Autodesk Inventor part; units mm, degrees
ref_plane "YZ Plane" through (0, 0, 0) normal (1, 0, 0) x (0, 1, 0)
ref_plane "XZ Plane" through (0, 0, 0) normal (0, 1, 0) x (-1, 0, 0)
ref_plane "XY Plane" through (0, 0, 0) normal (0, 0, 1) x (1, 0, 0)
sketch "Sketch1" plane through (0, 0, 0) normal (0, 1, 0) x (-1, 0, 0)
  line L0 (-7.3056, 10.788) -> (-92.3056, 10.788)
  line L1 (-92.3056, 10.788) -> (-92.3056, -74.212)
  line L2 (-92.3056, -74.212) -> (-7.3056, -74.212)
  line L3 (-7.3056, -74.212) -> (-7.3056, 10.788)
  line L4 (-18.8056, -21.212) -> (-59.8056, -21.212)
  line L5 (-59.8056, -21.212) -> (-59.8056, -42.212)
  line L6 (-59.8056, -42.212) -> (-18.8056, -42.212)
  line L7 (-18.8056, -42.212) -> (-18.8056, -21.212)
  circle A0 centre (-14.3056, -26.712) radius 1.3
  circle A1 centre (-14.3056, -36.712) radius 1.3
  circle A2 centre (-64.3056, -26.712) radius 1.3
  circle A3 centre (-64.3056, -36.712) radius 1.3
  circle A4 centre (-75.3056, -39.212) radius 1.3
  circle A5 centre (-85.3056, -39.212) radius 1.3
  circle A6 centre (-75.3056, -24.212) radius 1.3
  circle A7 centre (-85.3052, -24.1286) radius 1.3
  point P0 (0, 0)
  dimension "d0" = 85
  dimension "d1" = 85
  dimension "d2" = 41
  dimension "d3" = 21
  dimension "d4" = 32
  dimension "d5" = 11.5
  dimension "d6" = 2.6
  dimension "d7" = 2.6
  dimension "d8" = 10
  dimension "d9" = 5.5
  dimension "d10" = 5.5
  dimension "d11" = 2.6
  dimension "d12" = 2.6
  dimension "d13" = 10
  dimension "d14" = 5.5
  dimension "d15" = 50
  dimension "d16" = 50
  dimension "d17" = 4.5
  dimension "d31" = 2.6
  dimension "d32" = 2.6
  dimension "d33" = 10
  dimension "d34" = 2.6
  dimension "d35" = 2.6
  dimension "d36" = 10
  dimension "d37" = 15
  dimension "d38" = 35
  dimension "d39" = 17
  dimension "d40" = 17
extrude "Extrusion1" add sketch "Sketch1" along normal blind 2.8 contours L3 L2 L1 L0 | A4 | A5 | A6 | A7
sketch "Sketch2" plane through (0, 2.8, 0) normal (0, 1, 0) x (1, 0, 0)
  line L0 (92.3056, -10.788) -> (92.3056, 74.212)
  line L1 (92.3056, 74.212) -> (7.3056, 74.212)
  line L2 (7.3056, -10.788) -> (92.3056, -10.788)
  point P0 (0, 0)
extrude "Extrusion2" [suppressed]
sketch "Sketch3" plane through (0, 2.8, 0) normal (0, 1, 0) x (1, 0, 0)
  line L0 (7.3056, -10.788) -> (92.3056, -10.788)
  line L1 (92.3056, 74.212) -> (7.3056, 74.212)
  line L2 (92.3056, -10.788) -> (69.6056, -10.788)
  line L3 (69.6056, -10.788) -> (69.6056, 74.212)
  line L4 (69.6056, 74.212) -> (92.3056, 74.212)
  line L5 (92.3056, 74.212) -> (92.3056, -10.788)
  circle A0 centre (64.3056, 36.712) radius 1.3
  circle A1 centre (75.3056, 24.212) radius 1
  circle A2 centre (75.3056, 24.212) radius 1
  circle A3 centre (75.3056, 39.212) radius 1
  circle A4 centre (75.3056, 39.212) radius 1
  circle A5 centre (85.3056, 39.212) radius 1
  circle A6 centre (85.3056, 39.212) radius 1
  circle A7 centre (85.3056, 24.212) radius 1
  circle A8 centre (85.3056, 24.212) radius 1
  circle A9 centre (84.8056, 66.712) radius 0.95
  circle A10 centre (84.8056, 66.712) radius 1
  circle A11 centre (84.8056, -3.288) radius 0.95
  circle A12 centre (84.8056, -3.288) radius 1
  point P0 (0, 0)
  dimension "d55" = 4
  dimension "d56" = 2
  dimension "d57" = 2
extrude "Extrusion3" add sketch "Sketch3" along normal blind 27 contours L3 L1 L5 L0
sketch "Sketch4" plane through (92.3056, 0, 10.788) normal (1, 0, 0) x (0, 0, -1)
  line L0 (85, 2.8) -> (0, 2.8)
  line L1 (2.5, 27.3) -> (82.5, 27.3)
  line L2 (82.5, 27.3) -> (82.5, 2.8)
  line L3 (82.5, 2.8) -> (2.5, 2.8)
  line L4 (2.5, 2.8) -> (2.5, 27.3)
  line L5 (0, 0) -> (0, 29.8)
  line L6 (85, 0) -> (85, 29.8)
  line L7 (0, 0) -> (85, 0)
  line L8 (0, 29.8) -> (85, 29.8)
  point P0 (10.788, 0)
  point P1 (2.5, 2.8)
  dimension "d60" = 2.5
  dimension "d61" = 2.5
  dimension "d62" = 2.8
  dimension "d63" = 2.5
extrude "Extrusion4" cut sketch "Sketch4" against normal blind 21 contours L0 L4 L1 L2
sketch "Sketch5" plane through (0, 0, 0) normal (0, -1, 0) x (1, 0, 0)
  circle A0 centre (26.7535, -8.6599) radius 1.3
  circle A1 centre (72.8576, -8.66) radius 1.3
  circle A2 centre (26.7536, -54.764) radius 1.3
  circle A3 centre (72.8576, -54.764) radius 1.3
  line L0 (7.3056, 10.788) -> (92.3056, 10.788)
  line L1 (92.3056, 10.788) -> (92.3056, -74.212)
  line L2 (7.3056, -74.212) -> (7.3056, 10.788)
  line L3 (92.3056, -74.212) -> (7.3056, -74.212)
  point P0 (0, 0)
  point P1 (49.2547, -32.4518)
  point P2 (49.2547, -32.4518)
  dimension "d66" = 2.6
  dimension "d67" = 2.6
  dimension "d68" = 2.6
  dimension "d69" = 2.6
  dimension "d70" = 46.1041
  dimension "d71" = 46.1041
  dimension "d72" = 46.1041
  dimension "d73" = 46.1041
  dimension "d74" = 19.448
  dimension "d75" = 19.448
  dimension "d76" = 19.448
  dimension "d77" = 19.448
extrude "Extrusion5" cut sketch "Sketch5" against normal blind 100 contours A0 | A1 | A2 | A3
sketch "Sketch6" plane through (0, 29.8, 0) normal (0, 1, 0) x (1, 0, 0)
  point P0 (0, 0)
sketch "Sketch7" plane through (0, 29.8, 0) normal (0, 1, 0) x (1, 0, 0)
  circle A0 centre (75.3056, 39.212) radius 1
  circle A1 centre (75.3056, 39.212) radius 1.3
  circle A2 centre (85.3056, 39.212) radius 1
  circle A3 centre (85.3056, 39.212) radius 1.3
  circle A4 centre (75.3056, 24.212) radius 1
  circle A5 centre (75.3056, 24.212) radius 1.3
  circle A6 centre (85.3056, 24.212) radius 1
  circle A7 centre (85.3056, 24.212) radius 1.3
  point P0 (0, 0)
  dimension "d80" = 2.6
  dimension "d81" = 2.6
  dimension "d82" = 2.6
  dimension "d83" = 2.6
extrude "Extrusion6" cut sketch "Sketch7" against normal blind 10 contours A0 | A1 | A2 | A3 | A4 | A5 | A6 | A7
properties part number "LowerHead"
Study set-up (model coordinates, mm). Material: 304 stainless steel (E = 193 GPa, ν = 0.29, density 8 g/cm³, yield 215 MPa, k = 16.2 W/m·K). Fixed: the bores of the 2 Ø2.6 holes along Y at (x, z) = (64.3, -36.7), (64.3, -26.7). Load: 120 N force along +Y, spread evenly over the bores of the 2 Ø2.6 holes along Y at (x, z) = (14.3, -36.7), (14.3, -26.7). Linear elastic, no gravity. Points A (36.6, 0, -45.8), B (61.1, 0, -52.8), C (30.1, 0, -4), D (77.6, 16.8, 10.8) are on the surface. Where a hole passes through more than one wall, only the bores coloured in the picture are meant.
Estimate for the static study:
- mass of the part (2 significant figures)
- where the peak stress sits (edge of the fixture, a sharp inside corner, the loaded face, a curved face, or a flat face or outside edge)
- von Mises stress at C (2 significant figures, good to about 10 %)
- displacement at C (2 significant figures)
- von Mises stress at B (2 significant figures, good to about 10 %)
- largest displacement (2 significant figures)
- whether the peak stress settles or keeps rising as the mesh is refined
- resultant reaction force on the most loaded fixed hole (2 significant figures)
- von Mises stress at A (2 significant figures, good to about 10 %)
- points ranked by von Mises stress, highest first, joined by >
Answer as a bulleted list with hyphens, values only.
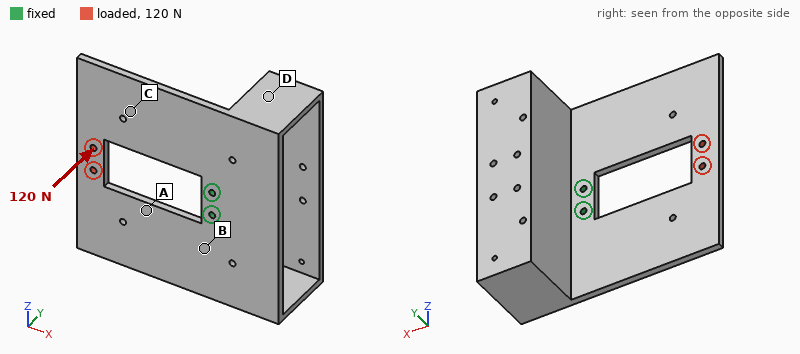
- 230 g
- edge of the fixture
- 27 MPa
- 0.26 mm
- 64 MPa
- 0.52 mm
- keeps rising
- 60 N
- 44 MPa
- B > A > C > D
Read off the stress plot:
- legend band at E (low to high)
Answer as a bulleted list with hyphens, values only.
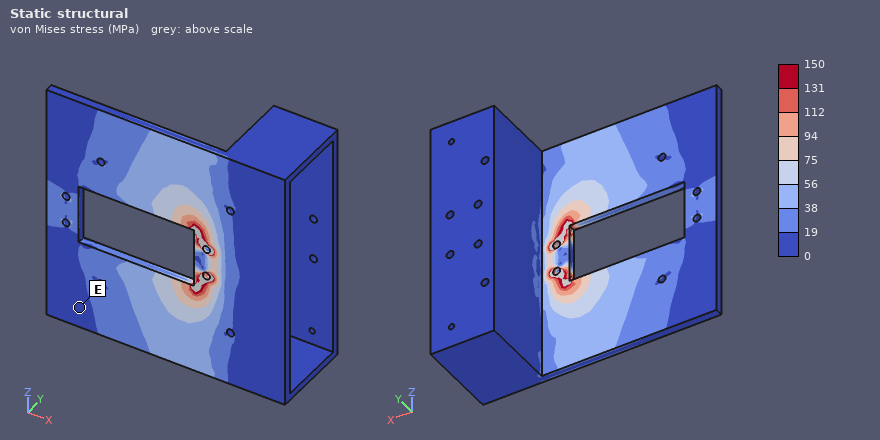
- 0 to 19 MPa
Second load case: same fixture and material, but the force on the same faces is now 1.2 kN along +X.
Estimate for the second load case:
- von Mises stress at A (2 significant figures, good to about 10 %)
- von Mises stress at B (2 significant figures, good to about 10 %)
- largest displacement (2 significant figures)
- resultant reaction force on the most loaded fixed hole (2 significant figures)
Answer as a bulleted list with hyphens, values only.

- 20 MPa
- 9.8 MPa
- 13 µm
- 650 N
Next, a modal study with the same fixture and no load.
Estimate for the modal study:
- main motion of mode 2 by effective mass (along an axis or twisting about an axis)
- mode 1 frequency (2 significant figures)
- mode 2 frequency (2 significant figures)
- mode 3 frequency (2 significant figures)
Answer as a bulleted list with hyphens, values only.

- twisting about X
- 400 Hz
- 810 Hz
- 880 Hz
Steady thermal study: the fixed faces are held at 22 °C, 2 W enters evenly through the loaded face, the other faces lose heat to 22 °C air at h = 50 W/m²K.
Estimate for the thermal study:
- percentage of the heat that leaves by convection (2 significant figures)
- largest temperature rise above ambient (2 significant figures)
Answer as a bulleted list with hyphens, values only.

- 98 %
- 27 K
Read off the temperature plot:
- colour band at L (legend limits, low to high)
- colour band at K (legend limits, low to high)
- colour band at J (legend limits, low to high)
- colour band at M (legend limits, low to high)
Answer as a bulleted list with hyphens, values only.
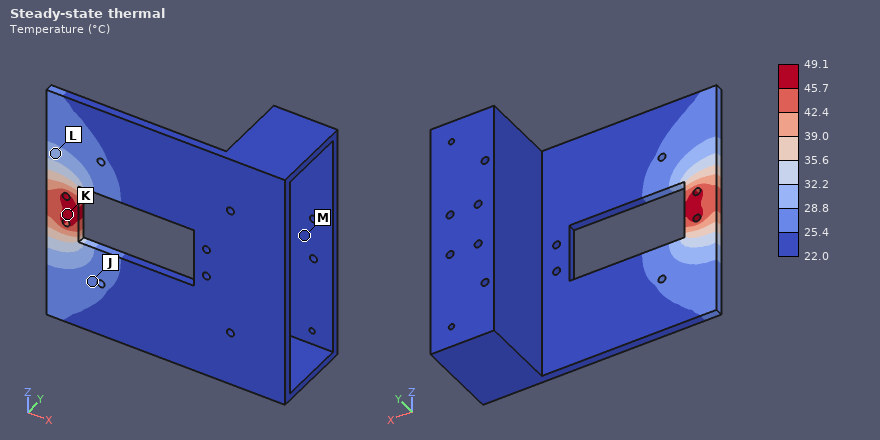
- 28.8 to 32.2 °C
- 45.7 to 49.1 °C
- 25.4 to 28.8 °C
- 22.0 to 25.4 °C
